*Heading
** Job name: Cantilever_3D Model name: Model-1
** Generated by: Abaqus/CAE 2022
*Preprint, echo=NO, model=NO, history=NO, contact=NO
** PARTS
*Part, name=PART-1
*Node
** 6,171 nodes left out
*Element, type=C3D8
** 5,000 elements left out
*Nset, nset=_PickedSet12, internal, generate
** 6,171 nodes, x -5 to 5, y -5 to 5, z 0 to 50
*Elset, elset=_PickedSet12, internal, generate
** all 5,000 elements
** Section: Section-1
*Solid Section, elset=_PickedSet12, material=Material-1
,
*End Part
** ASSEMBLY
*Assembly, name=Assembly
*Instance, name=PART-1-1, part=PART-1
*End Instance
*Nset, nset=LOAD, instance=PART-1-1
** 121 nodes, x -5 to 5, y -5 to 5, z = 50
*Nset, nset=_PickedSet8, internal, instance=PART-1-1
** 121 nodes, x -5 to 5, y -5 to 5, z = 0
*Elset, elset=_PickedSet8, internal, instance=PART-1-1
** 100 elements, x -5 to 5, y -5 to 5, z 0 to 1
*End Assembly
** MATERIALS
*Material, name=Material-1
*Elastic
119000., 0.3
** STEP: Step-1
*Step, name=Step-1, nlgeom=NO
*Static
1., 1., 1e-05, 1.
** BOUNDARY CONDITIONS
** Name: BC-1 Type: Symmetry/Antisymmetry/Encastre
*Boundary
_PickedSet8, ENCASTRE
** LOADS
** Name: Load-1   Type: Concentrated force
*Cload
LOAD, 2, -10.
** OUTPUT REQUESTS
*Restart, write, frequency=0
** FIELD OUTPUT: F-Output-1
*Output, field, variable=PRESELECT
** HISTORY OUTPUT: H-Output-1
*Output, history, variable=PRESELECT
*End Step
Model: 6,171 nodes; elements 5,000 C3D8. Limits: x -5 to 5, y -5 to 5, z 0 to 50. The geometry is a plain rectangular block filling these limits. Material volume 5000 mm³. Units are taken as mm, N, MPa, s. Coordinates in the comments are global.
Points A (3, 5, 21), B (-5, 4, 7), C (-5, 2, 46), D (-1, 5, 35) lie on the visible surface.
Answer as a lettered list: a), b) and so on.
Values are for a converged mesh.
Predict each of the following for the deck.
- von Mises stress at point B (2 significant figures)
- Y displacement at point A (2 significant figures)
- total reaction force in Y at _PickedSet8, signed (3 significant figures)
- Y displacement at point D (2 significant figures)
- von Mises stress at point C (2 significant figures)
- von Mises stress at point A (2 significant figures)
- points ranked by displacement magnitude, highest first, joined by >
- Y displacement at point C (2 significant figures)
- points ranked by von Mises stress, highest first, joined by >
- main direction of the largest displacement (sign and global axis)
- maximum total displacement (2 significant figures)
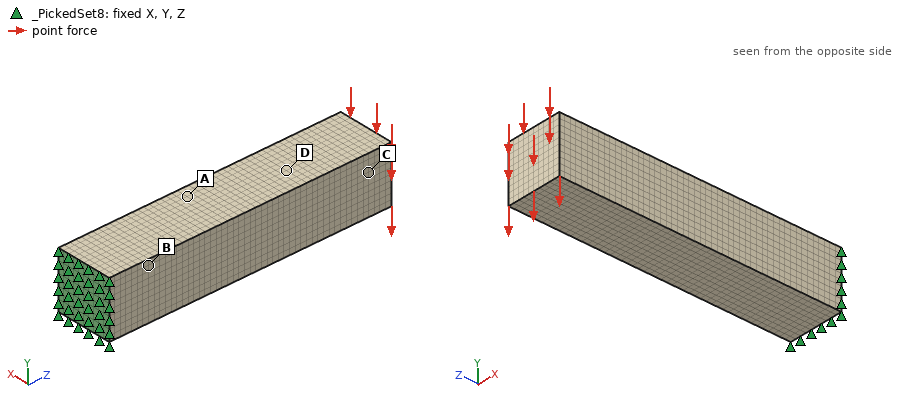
a) 240 MPa
b) -0.12 mm
c) 1210 N
d) -0.29 mm
e) 33 MPa
f) 210 MPa
g) C > D > A > B
h) -0.46 mm
i) B > A > D > C
j) -Y
k) 0.52 mm
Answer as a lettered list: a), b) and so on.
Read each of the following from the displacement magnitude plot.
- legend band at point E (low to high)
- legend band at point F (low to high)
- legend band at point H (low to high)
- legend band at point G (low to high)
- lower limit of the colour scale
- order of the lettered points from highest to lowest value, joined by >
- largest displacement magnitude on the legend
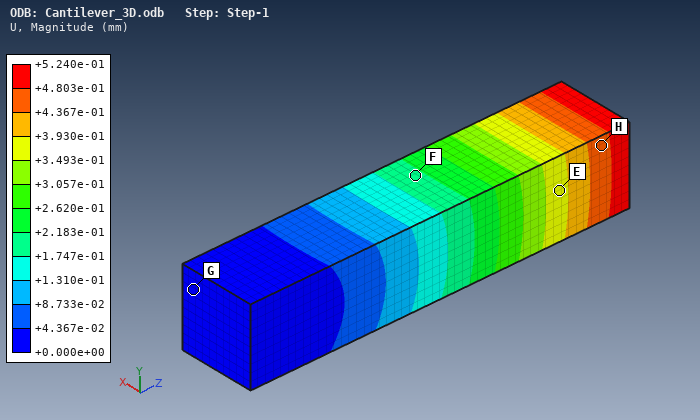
a) +3.493e-01 to +3.930e-01 mm
b) +1.747e-01 to +2.183e-01 mm
c) +4.367e-01 to +4.803e-01 mm
d) +0.000e+00 to +4.367e-02 mm
e) +0.000e+00 mm
f) H > E > F > G
g) +5.240e-01 mm
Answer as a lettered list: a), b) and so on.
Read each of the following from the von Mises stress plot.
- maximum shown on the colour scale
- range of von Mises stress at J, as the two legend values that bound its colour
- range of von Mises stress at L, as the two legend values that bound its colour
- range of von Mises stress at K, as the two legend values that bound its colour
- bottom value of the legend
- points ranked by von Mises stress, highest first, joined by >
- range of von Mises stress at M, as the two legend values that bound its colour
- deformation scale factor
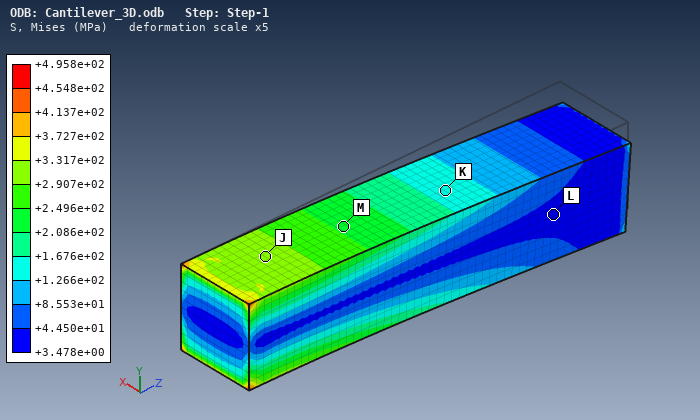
a) +4.958e+02 MPa
b) +2.907e+02 to +3.317e+02 MPa
c) +3.478e+00 to +4.450e+01 MPa
d) +1.266e+02 to +1.676e+02 MPa
e) +3.478e+00 MPa
f) J > M > K > L
g) +2.086e+02 to +2.496e+02 MPa
h) 5
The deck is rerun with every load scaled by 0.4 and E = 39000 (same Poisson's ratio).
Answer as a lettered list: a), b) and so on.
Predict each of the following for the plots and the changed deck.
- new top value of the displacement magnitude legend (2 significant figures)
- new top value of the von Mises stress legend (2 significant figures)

a) 0.64 mm
b) 200 MPa
